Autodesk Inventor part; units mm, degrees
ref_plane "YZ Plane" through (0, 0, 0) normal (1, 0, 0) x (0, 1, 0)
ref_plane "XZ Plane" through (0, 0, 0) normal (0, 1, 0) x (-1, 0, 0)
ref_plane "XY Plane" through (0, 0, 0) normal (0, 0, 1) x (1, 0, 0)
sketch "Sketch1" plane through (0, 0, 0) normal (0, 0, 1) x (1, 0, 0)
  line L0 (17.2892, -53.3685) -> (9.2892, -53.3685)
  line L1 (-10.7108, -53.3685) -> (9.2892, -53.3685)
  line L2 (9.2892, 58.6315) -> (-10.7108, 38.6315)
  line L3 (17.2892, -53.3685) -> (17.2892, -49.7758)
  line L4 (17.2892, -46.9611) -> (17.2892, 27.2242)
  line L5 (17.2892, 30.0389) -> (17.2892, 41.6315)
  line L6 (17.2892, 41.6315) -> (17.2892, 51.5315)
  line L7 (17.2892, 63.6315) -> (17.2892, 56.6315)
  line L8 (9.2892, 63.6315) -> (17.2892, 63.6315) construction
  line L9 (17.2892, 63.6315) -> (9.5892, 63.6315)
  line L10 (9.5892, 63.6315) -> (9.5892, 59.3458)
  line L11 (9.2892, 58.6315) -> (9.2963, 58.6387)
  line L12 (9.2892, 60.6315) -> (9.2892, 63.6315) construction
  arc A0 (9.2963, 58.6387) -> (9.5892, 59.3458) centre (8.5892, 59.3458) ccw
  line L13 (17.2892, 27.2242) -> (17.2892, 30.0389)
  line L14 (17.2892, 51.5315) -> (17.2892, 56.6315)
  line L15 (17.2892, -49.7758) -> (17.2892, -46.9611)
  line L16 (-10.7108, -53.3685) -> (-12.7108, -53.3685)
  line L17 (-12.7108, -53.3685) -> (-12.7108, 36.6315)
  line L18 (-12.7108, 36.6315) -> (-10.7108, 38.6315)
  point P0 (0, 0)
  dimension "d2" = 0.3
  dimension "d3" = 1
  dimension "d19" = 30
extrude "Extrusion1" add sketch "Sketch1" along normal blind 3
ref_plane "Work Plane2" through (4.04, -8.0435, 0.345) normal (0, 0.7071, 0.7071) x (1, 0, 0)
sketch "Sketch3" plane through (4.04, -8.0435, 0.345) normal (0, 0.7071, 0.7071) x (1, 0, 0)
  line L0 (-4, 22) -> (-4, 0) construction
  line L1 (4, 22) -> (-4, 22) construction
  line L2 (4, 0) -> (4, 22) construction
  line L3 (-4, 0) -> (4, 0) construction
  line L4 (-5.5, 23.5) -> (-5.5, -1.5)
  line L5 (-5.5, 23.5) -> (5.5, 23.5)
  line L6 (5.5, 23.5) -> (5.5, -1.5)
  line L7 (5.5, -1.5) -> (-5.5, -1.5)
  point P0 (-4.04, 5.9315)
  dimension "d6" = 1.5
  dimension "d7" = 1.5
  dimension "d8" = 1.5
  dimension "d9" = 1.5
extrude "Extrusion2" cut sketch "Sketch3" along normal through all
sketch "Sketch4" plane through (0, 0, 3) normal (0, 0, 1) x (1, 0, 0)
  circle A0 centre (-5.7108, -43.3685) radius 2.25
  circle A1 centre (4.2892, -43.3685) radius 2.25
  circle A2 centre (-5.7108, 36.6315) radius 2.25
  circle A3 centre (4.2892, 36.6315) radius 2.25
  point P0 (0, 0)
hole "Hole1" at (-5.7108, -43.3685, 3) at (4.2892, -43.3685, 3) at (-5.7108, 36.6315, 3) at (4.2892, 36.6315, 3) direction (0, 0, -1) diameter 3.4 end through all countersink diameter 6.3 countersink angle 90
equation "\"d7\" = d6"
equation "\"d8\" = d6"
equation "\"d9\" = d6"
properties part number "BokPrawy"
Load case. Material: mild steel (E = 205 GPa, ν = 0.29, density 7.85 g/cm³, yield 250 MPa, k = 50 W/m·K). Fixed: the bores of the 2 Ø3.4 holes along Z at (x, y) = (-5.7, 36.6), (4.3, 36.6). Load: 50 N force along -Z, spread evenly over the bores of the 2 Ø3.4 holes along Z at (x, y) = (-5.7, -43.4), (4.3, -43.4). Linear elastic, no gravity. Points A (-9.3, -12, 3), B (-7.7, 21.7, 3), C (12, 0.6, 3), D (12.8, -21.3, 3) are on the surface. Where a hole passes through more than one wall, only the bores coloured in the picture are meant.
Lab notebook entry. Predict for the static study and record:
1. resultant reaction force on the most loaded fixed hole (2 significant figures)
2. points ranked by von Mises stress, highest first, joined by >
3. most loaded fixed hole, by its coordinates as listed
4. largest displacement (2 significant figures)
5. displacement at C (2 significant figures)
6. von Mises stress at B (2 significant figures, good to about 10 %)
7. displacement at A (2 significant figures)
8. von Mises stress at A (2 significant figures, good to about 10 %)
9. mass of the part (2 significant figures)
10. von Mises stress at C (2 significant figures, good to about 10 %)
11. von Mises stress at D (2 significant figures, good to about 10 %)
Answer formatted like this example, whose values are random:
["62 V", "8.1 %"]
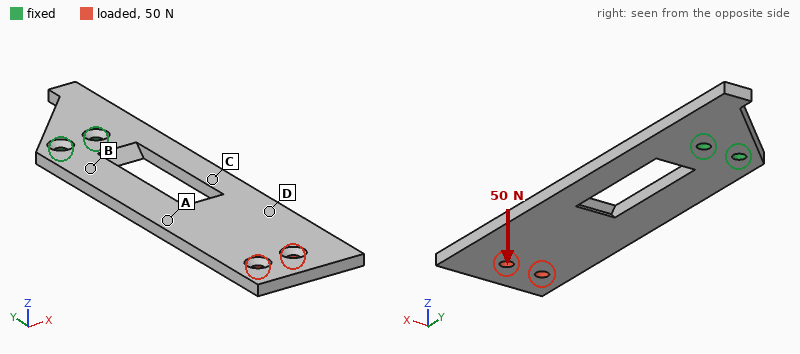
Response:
["50 N", "B > C > A > D", "(-5.7, 36.6)", "1.1 mm", "0.24 mm", "110 MPa", "0.43 mm", "44 MPa", "64 g", "79 MPa", "24 MPa"]
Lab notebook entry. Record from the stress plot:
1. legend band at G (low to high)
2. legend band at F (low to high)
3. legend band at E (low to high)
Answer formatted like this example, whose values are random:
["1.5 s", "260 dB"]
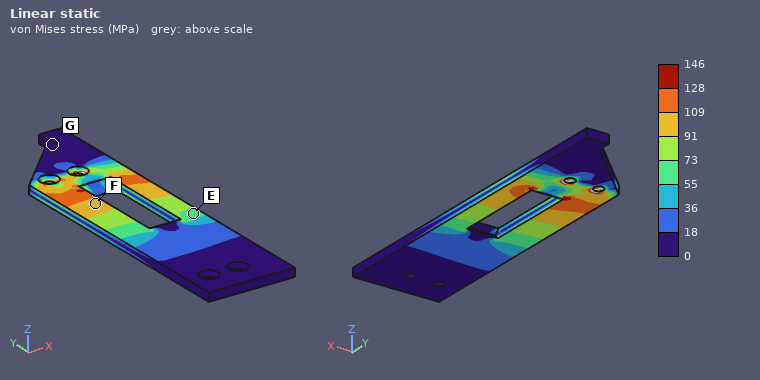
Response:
["0 to 18 MPa", "91 to 109 MPa", "55 to 73 MPa"]
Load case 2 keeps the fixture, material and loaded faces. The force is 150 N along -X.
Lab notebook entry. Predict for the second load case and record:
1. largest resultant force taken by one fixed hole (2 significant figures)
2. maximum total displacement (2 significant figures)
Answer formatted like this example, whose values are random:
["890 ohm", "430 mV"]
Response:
["970 N", "57 µm"]
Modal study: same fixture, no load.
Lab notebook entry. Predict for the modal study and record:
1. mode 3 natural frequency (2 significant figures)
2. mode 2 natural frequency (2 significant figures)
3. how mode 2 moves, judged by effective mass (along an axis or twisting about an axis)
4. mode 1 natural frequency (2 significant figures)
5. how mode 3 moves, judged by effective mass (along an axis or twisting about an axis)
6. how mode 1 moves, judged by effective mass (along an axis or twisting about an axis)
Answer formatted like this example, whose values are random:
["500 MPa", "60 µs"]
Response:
["1800 Hz", "1500 Hz", "twisting about Y", "250 Hz", "along X", "along Z"]
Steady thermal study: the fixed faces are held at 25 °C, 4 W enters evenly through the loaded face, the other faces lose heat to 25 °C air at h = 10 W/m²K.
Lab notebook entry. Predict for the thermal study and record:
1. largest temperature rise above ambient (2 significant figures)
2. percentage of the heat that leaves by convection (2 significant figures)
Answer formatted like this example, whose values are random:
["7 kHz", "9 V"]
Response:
["64 K", "48 %"]
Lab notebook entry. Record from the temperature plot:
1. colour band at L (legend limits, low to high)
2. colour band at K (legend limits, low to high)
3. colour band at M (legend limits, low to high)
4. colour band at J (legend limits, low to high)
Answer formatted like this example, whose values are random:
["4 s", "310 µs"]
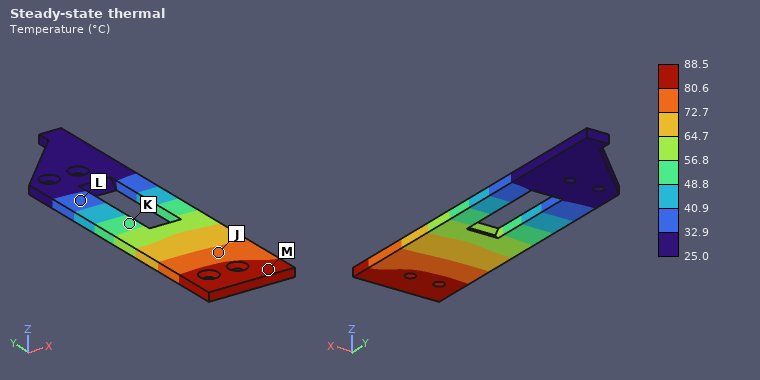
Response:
["32.9 to 40.9 °C", "48.8 to 56.8 °C", "80.6 to 88.5 °C", "72.7 to 80.6 °C"]
